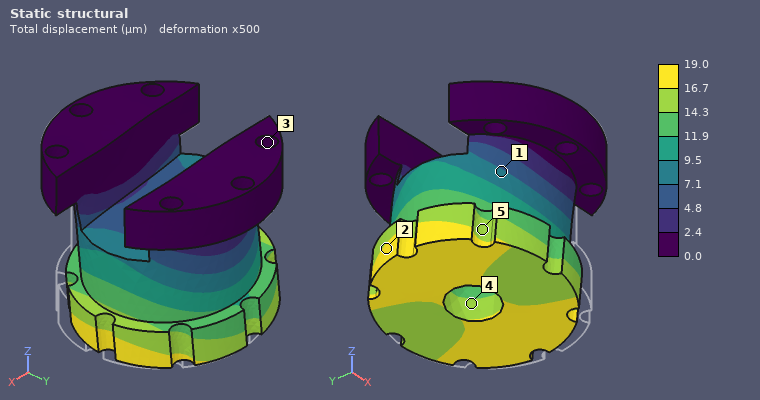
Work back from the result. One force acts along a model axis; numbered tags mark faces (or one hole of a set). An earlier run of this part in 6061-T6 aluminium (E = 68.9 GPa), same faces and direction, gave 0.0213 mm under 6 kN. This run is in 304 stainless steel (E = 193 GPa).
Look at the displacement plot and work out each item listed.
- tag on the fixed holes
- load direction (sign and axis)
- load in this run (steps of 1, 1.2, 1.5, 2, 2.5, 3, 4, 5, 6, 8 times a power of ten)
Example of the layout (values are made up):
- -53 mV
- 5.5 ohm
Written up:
- 3
- -X
- 15 kN
